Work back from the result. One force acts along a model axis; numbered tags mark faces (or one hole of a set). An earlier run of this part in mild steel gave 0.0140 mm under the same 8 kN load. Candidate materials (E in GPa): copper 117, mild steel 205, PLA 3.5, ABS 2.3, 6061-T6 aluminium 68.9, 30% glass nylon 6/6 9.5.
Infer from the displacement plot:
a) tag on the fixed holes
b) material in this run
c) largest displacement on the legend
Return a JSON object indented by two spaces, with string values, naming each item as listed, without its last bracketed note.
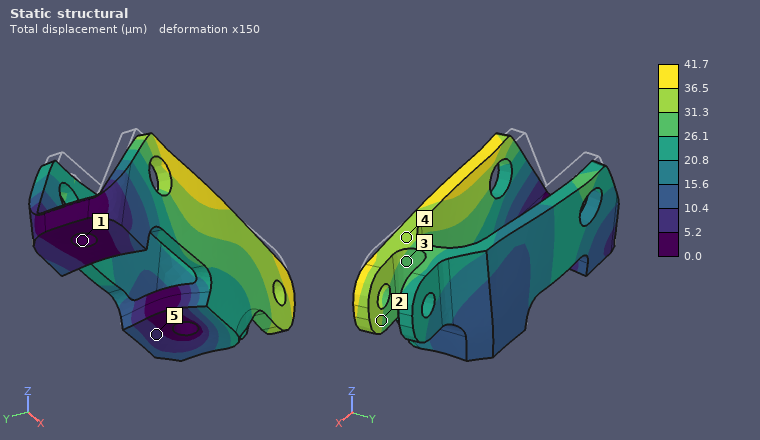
{
  "tag on the fixed holes": "1",
  "material in this run": "6061-T6 aluminium",
  "largest displacement on the legend": "41.7 µm"
}
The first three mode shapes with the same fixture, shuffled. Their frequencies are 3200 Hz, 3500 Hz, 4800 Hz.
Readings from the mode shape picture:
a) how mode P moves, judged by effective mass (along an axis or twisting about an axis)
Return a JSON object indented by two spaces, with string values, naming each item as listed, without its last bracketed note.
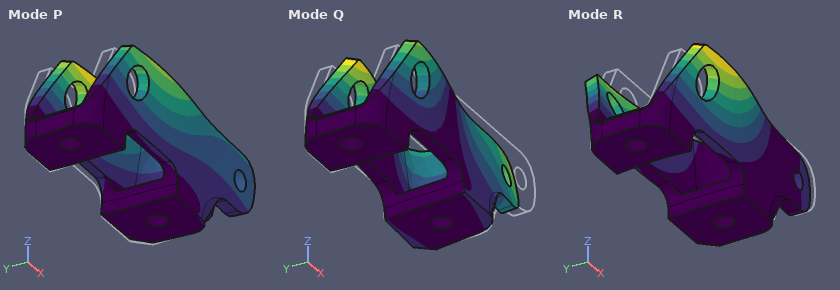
{
  "how mode P moves, judged by effective mass": "along Y"
}
